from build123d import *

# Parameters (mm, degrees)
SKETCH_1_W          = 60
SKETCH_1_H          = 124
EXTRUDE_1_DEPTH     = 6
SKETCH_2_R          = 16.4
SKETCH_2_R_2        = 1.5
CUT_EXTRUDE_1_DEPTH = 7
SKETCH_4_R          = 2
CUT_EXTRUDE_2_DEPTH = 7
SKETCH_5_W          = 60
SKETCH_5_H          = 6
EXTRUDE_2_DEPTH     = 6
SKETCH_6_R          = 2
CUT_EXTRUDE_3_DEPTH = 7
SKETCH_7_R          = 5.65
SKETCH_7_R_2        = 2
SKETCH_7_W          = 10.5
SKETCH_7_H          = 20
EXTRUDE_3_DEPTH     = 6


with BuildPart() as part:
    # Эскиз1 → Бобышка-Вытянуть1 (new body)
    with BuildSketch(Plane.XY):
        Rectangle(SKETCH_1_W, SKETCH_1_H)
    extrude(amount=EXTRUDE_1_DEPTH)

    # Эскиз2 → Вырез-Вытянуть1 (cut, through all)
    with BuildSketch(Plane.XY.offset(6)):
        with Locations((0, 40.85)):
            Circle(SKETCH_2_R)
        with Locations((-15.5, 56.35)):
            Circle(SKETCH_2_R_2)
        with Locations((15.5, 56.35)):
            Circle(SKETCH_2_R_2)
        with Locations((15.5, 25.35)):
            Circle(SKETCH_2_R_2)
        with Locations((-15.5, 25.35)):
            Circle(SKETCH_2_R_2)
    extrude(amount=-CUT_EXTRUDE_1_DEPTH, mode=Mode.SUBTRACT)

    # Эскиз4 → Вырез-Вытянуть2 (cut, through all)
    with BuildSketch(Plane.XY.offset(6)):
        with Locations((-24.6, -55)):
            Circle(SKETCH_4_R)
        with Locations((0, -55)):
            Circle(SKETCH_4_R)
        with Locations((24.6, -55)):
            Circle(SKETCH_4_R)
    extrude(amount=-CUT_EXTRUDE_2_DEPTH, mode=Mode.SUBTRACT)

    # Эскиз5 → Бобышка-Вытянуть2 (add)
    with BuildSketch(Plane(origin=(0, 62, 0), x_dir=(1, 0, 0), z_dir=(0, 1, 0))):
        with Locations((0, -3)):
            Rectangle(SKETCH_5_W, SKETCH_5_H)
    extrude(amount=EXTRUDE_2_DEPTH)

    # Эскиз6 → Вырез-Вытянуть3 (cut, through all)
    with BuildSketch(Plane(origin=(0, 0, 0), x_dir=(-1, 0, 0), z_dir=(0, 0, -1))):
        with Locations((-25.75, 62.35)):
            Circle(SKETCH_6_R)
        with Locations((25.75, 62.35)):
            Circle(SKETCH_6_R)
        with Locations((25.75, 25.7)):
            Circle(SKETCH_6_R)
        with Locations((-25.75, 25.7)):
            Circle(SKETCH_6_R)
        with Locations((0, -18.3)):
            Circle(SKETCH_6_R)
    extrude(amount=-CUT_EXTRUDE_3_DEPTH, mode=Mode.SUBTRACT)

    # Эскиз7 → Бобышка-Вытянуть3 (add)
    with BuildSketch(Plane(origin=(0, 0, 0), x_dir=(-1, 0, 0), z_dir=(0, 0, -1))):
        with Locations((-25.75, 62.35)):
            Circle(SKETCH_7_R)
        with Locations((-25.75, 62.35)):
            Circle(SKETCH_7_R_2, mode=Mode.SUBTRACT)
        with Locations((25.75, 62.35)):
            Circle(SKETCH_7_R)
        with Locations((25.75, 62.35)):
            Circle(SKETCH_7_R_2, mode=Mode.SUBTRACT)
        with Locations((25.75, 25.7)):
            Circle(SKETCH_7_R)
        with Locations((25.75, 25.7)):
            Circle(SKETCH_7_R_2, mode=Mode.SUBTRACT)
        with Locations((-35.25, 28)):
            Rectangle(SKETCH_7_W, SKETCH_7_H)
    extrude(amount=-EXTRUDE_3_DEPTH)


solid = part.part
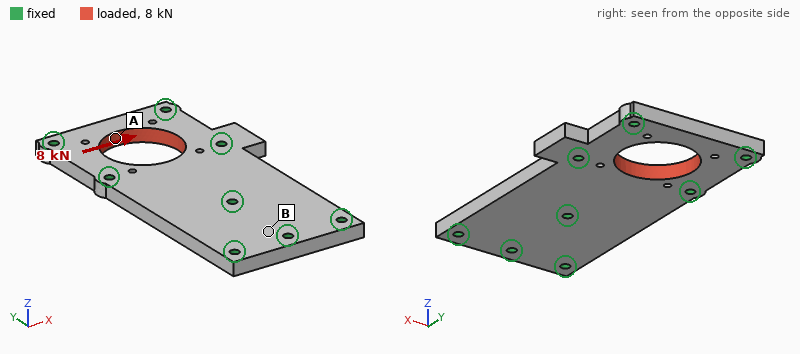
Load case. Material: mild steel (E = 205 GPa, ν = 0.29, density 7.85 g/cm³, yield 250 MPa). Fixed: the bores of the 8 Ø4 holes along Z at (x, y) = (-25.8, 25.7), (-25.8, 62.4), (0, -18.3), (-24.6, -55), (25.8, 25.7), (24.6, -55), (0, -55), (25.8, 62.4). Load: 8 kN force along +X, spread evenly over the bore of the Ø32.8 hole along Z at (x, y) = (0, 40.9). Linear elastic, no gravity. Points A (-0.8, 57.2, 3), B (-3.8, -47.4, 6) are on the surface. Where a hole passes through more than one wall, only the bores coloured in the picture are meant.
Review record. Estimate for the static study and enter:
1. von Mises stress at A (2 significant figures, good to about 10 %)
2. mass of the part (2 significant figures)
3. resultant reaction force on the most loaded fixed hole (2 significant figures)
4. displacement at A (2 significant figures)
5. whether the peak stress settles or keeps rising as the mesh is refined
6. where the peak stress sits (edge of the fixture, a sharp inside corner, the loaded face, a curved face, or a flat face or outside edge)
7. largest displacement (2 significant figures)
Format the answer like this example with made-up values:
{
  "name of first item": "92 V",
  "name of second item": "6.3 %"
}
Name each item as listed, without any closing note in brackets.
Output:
{
  "von Mises stress at A": "22 MPa",
  "mass of the part": "330 g",
  "resultant reaction force on the most loaded fixed hole": "2.2 kN",
  "displacement at A": "2.1 µm",
  "whether the peak stress settles or keeps rising as the mesh is refined": "keeps rising",
  "where the peak stress sits": "edge of the fixture",
  "largest displacement": "3.2 µm"
}
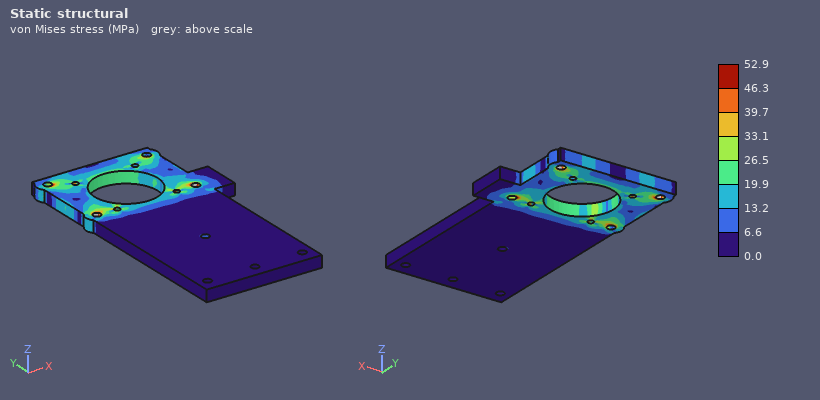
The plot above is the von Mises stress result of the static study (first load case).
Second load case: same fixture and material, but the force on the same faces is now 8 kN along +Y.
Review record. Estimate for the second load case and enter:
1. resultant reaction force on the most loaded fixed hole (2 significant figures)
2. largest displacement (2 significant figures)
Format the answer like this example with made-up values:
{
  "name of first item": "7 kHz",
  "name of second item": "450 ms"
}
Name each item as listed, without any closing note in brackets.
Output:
{
  "resultant reaction force on the most loaded fixed hole": "2.0 kN",
  "largest displacement": "7.0 µm"
}
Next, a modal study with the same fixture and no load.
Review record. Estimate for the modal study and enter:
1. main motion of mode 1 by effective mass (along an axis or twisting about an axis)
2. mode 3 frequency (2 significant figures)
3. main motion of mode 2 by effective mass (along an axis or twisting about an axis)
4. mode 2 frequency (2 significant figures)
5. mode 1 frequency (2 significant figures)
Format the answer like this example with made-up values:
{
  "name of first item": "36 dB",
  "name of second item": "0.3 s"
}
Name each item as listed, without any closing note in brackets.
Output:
{
  "main motion of mode 1 by effective mass": "twisting about Y",
  "mode 3 frequency": "11 kHz",
  "main motion of mode 2 by effective mass": "along Z",
  "mode 2 frequency": "8100 Hz",
  "mode 1 frequency": "7300 Hz"
}
